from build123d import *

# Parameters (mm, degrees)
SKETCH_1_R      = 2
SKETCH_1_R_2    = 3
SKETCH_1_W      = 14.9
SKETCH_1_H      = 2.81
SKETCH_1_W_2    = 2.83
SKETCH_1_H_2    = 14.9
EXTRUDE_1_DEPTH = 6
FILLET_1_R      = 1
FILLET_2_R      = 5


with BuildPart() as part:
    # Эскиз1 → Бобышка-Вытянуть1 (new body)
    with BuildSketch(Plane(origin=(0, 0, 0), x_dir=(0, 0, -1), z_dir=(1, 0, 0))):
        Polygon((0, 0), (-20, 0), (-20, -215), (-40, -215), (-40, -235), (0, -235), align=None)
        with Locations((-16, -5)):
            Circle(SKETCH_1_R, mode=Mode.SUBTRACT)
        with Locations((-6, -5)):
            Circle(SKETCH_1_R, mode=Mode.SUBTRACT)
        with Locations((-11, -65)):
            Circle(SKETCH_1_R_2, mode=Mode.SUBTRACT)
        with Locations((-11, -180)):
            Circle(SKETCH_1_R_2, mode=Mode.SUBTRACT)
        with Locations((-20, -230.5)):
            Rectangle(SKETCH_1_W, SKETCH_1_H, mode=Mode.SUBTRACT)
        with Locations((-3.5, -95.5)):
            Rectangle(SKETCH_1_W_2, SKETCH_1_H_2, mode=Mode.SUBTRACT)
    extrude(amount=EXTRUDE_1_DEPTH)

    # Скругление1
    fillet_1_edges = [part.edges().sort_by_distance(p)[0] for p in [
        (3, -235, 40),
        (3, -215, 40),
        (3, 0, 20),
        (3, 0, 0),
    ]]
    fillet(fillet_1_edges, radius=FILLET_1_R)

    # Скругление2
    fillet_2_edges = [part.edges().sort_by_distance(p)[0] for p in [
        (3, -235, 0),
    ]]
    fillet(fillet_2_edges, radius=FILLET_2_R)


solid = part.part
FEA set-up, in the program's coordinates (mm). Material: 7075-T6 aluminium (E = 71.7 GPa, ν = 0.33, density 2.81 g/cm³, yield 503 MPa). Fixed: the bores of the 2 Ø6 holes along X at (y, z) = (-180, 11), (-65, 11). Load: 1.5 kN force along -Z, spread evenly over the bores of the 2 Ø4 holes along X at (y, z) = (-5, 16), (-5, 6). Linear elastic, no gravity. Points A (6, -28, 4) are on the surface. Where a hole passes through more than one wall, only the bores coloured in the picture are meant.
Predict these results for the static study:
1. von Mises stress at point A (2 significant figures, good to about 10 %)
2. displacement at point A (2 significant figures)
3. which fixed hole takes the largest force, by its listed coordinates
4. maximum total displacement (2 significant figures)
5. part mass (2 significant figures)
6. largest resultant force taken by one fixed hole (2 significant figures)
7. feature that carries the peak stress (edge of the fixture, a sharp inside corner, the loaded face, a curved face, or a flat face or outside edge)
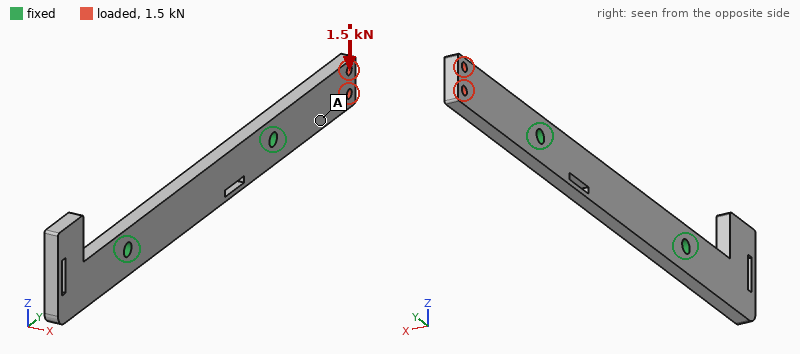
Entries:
57 MPa
0.30 mm
(-65, 11)
0.65 mm
83 g
1.8 kN
edge of the fixture
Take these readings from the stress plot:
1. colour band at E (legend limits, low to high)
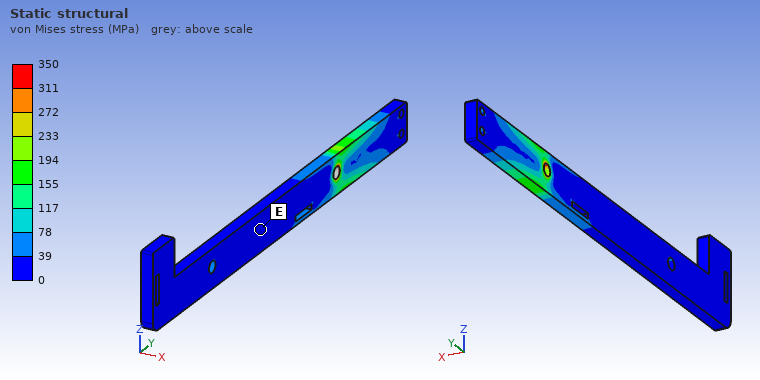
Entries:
0 to 39 MPa
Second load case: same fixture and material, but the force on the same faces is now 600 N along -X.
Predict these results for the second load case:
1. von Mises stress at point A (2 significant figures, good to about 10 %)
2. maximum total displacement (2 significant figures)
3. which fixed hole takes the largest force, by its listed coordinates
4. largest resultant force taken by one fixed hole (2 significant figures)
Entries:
120 MPa
1.8 mm
(-65, 11)
610 N
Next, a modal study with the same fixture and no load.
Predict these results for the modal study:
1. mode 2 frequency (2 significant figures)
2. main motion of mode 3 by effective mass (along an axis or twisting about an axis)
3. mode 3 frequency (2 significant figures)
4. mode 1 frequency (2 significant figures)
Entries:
1200 Hz
along X
2400 Hz
1200 Hz
